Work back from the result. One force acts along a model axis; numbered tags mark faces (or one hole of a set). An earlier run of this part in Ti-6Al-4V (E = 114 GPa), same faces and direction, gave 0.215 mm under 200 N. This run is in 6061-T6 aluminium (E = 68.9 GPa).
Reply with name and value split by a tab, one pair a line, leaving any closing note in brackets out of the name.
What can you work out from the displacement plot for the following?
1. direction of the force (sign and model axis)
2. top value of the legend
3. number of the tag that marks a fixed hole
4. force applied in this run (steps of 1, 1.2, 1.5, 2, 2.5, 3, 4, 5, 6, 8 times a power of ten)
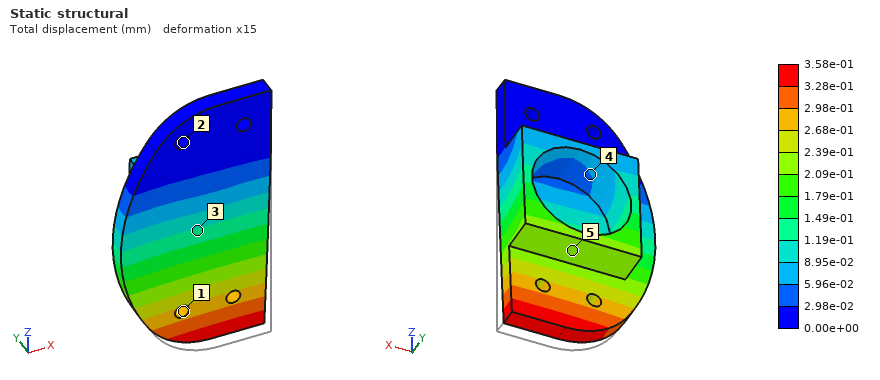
direction of the force	+Y
top value of the legend	3.58e-01 mm
number of the tag that marks a fixed hole	2
force applied in this run	200 N
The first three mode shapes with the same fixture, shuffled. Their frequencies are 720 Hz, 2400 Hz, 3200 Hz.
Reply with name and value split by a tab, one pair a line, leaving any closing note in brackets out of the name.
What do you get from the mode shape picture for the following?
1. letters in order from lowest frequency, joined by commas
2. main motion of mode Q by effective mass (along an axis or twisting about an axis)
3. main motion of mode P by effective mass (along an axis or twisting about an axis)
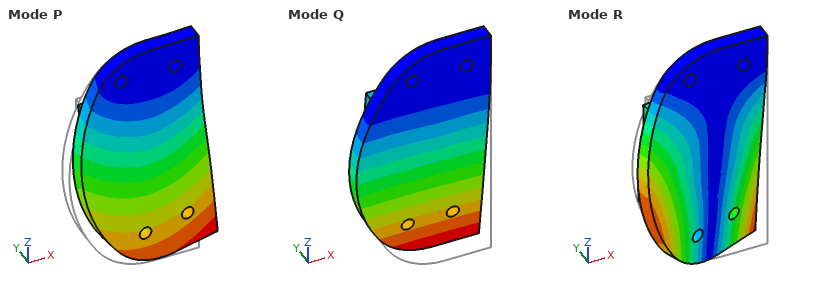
letters in order from lowest frequency, joined by commas	Q, R, P
main motion of mode Q by effective mass	along Y
main motion of mode P by effective mass	along X
